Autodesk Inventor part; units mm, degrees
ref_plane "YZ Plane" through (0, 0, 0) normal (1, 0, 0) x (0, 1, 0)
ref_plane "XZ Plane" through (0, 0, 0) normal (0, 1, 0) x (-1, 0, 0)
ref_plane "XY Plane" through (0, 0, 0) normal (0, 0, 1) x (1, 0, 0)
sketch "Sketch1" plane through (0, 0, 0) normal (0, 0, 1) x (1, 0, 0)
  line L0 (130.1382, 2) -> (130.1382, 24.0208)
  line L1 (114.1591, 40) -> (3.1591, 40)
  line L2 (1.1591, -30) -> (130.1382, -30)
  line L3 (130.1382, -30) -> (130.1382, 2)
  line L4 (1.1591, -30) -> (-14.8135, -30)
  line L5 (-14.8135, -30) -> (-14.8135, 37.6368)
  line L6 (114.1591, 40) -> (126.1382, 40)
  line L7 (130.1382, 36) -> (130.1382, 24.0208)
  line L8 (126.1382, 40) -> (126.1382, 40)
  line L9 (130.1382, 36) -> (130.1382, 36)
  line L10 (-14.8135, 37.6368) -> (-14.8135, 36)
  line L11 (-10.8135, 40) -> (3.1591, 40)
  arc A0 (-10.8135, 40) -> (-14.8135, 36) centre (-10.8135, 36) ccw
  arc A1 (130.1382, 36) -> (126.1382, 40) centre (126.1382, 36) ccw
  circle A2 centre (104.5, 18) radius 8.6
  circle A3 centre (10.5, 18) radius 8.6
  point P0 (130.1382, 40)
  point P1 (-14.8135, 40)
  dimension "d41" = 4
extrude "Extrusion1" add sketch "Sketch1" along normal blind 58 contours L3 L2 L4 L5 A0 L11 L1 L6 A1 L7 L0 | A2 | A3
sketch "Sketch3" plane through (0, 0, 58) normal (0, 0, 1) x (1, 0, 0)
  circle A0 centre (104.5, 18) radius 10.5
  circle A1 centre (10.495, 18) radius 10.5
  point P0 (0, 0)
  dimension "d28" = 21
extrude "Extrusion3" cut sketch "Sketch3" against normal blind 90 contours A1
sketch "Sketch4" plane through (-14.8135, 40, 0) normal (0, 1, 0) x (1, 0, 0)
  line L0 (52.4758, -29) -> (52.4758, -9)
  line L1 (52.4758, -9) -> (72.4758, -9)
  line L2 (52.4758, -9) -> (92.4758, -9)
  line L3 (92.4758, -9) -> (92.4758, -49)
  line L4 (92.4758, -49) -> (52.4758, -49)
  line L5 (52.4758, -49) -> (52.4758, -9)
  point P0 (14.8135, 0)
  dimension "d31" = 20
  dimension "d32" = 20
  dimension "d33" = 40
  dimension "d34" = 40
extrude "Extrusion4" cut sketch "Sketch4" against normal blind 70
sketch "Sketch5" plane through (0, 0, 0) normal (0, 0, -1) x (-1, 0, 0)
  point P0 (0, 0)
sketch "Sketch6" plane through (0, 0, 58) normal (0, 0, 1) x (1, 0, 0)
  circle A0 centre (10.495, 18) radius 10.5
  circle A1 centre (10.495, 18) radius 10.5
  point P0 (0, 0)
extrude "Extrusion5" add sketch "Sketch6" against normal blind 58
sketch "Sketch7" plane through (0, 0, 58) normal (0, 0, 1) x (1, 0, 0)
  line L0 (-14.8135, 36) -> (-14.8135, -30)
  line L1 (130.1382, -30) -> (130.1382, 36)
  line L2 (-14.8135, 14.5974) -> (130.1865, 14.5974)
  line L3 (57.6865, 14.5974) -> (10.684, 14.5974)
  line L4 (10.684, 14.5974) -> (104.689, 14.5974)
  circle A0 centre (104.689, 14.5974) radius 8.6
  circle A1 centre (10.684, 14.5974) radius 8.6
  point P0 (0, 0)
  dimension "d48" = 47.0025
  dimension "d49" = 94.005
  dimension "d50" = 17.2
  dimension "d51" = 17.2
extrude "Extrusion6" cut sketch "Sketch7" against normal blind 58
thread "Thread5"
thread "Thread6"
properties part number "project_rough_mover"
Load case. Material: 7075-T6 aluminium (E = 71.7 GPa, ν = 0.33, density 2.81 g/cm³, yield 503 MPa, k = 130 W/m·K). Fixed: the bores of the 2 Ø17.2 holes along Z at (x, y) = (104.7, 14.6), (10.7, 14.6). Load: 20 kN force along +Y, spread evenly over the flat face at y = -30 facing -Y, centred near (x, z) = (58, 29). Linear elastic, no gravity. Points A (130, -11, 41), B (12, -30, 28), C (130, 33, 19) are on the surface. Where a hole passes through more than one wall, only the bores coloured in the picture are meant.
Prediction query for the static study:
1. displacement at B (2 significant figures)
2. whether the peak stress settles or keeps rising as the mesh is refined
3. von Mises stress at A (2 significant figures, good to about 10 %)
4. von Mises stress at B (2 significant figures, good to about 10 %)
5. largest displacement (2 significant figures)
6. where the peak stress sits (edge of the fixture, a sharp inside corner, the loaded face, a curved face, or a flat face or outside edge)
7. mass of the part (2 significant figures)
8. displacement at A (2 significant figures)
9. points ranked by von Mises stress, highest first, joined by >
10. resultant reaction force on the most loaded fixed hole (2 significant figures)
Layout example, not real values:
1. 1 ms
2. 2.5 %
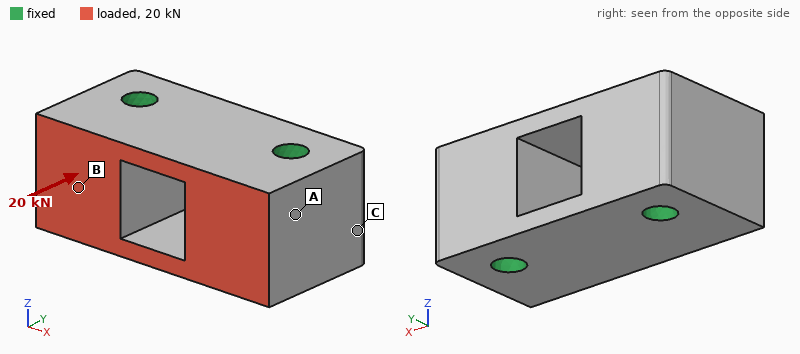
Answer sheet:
1. 1.9 µm
2. keeps rising
3. 2.2 MPa
4. 3.5 MPa
5. 3.0 µm
6. edge of the fixture
7. 1.3 kg
8. 1.3 µm
9. B > A > C
10. 10 kN
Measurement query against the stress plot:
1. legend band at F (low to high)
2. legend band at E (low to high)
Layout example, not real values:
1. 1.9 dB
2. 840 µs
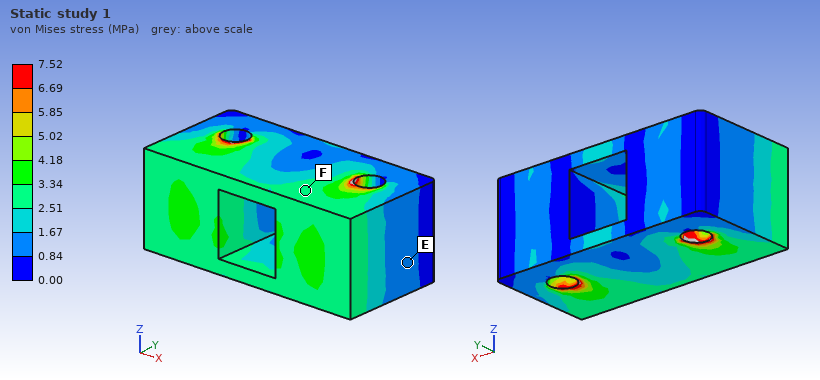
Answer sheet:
1. 2.51 to 3.34 MPa
2. 0.84 to 1.67 MPa
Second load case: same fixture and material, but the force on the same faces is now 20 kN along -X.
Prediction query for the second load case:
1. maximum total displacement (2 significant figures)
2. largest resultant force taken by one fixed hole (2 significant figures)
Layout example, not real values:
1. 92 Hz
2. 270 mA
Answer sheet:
1. 13 µm
2. 11 kN
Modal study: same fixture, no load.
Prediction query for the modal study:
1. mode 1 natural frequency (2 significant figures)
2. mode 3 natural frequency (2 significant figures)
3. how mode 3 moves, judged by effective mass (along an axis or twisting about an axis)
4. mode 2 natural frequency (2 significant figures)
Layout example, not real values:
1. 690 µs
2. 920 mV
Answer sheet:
1. 12 kHz
2. 12 kHz
3. along X
4. 12 kHz
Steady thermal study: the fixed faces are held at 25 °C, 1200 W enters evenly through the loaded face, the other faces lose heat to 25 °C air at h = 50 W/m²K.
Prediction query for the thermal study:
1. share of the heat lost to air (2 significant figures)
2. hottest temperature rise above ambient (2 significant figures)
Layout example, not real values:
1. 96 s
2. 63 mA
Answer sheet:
1. 3.8 %
2. 62 K
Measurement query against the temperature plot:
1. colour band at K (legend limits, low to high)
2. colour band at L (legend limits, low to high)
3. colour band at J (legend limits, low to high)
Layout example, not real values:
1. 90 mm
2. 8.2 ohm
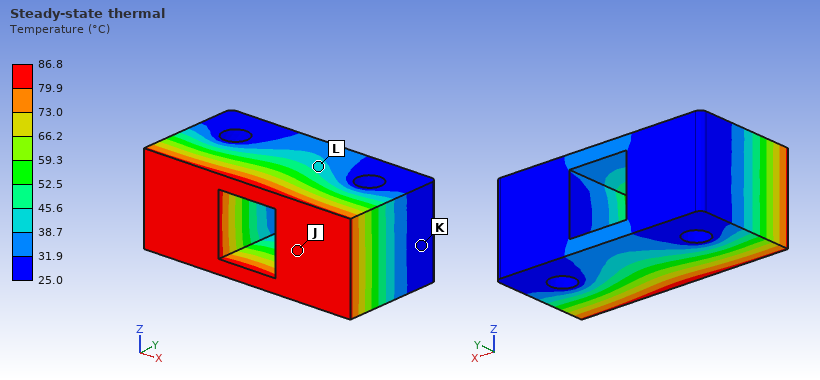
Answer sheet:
1. 25.0 to 31.9 °C
2. 38.7 to 45.6 °C
3. 79.9 to 86.8 °C
